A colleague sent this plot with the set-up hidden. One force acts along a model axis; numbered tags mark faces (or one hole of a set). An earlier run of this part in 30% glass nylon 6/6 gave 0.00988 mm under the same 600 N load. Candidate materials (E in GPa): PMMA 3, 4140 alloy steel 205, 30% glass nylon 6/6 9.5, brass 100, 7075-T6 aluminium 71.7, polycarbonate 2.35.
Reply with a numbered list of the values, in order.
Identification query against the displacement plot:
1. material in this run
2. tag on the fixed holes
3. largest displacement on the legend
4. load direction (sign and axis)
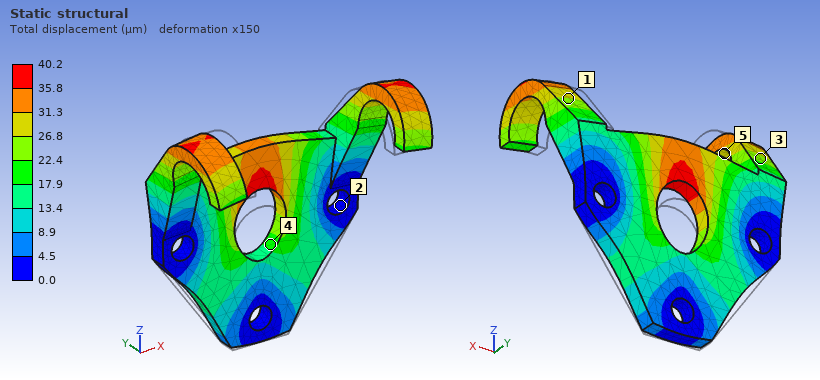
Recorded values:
1. polycarbonate
2. 2
3. 40.2 µm
4. +Z
